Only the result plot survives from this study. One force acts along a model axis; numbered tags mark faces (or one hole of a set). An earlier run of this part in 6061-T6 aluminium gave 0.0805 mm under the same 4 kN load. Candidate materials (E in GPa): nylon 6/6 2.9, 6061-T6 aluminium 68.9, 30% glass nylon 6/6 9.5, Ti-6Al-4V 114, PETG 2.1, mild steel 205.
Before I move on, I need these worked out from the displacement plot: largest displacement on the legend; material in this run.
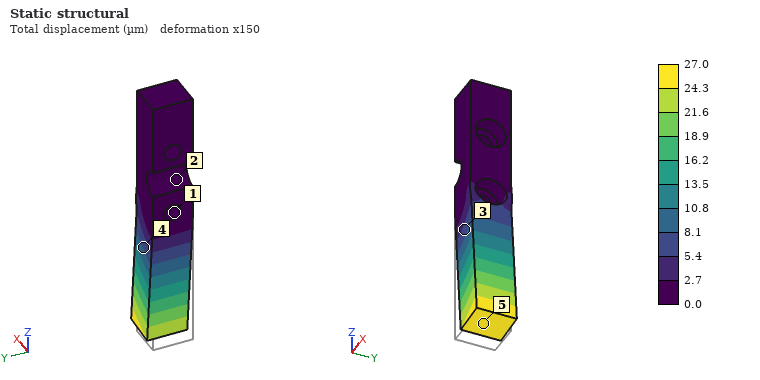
27.0 µm
mild steel
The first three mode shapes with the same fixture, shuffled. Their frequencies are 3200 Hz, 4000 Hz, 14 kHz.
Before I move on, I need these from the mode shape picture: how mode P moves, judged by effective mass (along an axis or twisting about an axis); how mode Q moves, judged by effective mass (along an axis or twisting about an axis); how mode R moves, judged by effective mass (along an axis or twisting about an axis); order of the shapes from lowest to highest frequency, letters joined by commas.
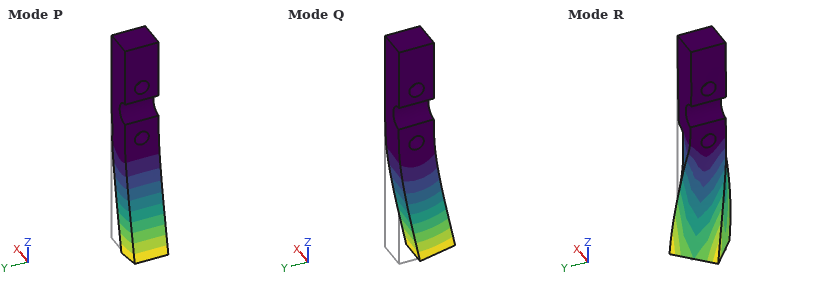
along X
along Y
twisting about Z
P, Q, R
